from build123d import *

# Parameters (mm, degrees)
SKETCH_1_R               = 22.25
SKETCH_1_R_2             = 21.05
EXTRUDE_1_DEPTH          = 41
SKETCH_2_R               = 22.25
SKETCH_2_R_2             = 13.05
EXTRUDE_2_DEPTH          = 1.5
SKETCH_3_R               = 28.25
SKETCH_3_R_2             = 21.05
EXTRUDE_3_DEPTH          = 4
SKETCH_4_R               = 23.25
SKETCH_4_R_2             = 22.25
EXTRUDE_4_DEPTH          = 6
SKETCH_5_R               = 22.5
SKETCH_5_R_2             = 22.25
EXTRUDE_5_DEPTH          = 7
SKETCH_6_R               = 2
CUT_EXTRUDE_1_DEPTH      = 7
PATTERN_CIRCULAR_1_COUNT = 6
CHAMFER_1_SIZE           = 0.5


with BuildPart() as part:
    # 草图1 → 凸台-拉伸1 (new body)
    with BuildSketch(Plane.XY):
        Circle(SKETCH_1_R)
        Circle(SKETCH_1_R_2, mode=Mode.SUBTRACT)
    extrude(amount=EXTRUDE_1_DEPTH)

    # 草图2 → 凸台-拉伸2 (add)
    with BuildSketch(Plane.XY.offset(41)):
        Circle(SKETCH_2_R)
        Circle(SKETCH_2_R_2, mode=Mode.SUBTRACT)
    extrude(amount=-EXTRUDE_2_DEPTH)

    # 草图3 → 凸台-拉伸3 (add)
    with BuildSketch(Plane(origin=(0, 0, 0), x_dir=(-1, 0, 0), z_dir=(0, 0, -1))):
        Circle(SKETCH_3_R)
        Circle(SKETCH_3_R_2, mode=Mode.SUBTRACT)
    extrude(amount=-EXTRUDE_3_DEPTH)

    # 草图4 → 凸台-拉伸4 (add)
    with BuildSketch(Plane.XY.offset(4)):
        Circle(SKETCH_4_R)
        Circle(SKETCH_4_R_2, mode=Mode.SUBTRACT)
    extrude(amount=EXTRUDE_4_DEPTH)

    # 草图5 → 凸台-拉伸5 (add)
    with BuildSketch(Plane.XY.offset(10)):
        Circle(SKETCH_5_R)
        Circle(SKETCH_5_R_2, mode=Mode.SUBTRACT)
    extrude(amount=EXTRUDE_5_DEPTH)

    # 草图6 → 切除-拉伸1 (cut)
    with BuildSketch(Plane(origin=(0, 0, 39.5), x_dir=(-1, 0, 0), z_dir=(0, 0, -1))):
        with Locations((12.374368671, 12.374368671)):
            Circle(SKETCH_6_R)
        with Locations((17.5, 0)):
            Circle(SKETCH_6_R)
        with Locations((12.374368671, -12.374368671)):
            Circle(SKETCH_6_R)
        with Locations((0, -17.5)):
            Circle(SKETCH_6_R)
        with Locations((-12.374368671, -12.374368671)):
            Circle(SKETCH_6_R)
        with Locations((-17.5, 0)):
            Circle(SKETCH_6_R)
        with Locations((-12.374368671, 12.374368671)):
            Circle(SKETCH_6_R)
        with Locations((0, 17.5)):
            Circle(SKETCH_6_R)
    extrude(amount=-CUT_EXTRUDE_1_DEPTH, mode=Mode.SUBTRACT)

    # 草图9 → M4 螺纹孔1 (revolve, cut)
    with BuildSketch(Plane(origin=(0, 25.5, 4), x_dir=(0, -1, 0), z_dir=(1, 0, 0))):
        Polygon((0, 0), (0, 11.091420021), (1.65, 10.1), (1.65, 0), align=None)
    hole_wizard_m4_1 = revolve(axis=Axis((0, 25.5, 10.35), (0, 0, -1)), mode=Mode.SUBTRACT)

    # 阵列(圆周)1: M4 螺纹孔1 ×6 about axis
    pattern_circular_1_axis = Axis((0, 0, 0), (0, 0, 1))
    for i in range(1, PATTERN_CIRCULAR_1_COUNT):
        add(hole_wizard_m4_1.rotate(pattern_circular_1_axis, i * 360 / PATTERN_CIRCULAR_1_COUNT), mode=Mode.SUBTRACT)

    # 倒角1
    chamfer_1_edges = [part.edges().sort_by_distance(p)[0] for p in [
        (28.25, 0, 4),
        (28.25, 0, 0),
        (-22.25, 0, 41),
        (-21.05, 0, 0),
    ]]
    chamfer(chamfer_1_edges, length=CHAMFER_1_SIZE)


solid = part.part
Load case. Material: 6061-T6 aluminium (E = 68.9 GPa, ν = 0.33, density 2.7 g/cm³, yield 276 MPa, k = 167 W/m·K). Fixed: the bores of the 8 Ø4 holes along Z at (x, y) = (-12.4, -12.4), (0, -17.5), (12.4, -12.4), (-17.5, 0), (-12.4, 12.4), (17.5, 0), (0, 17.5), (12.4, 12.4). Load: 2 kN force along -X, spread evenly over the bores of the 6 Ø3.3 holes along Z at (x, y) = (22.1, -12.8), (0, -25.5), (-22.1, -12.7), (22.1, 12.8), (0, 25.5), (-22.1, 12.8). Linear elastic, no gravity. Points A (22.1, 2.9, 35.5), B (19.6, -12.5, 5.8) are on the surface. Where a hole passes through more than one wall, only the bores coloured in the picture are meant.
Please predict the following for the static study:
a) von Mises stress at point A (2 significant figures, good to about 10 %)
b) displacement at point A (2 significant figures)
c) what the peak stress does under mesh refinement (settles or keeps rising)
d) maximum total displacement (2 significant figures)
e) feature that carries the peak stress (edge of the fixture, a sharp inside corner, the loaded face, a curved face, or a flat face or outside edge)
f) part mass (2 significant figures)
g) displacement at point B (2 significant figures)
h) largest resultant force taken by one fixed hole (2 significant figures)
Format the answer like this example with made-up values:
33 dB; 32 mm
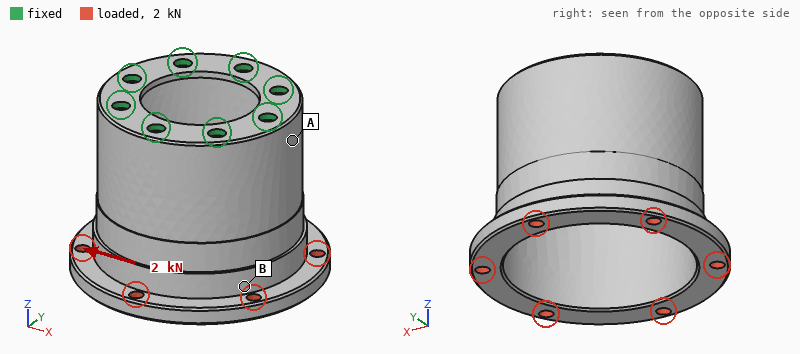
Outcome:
57 MPa; 0.041 mm; keeps rising; 0.12 mm; edge of the fixture; 34 g; 0.10 mm; 910 N
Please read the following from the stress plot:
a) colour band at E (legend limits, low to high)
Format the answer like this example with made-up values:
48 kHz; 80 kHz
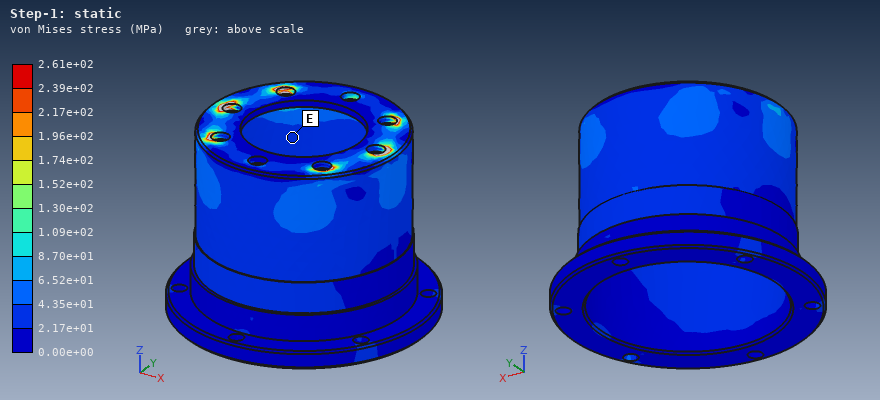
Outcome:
2.17e+01 to 4.35e+01 MPa
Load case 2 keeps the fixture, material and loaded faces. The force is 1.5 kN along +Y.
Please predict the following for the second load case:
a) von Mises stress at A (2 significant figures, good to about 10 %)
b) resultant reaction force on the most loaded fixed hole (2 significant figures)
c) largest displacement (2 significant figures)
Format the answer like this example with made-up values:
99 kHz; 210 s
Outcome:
30 MPa; 680 N; 95 µm
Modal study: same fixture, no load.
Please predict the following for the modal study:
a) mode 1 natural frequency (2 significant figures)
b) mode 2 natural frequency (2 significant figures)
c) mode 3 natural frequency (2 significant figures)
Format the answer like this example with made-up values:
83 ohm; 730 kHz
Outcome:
4800 Hz; 4800 Hz; 5900 Hz
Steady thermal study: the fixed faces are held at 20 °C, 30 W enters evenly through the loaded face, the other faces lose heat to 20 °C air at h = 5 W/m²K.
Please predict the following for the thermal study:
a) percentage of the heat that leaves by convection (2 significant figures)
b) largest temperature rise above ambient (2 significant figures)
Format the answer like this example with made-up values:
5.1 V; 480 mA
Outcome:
5.6 %; 42 K
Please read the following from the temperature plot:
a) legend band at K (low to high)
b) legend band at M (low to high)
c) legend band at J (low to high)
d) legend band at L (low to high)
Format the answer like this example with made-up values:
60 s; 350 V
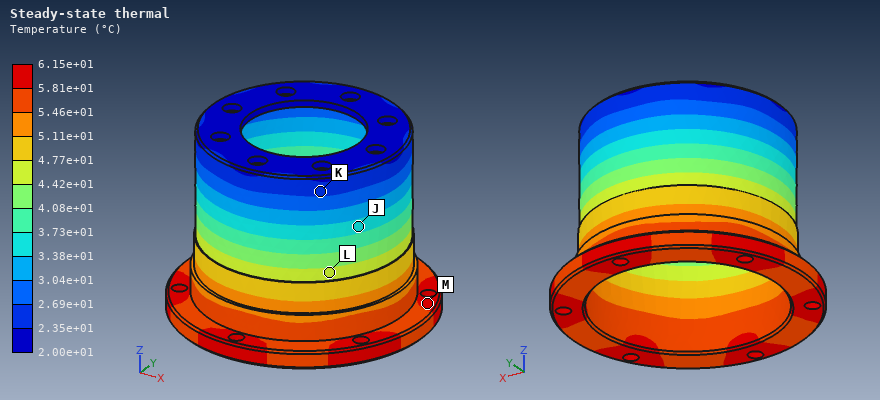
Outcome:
2.35e+01 to 2.69e+01 °C; 5.81e+01 to 6.15e+01 °C; 3.38e+01 to 3.73e+01 °C; 4.42e+01 to 4.77e+01 °C
